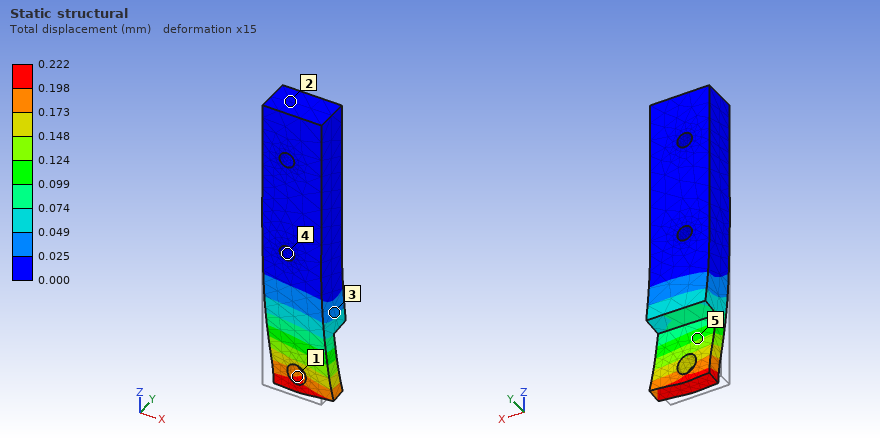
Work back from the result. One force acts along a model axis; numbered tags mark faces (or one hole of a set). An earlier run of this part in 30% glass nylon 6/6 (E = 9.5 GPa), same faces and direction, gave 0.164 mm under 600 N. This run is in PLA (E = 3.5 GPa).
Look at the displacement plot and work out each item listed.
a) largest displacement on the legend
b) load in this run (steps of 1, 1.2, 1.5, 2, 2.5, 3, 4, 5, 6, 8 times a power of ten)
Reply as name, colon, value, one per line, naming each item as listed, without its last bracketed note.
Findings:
largest displacement on the legend: 0.222 mm
load in this run: 300 N
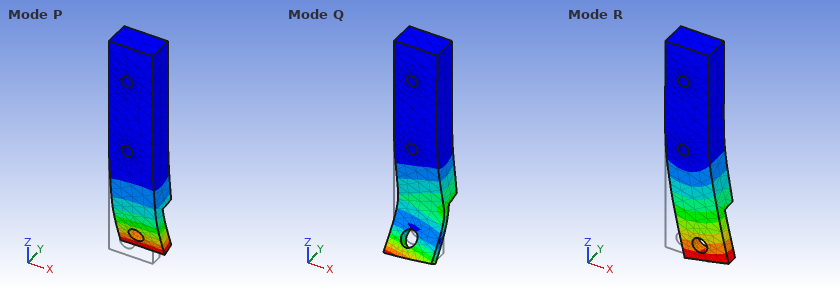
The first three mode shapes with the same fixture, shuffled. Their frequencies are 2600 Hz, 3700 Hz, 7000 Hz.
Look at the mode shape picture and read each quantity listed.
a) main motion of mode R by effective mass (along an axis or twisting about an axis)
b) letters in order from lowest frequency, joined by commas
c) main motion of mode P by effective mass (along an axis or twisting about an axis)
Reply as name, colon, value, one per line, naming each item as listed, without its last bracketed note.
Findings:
main motion of mode R by effective mass: along X
letters in order from lowest frequency, joined by commas: P, R, Q
main motion of mode P by effective mass: along Y
